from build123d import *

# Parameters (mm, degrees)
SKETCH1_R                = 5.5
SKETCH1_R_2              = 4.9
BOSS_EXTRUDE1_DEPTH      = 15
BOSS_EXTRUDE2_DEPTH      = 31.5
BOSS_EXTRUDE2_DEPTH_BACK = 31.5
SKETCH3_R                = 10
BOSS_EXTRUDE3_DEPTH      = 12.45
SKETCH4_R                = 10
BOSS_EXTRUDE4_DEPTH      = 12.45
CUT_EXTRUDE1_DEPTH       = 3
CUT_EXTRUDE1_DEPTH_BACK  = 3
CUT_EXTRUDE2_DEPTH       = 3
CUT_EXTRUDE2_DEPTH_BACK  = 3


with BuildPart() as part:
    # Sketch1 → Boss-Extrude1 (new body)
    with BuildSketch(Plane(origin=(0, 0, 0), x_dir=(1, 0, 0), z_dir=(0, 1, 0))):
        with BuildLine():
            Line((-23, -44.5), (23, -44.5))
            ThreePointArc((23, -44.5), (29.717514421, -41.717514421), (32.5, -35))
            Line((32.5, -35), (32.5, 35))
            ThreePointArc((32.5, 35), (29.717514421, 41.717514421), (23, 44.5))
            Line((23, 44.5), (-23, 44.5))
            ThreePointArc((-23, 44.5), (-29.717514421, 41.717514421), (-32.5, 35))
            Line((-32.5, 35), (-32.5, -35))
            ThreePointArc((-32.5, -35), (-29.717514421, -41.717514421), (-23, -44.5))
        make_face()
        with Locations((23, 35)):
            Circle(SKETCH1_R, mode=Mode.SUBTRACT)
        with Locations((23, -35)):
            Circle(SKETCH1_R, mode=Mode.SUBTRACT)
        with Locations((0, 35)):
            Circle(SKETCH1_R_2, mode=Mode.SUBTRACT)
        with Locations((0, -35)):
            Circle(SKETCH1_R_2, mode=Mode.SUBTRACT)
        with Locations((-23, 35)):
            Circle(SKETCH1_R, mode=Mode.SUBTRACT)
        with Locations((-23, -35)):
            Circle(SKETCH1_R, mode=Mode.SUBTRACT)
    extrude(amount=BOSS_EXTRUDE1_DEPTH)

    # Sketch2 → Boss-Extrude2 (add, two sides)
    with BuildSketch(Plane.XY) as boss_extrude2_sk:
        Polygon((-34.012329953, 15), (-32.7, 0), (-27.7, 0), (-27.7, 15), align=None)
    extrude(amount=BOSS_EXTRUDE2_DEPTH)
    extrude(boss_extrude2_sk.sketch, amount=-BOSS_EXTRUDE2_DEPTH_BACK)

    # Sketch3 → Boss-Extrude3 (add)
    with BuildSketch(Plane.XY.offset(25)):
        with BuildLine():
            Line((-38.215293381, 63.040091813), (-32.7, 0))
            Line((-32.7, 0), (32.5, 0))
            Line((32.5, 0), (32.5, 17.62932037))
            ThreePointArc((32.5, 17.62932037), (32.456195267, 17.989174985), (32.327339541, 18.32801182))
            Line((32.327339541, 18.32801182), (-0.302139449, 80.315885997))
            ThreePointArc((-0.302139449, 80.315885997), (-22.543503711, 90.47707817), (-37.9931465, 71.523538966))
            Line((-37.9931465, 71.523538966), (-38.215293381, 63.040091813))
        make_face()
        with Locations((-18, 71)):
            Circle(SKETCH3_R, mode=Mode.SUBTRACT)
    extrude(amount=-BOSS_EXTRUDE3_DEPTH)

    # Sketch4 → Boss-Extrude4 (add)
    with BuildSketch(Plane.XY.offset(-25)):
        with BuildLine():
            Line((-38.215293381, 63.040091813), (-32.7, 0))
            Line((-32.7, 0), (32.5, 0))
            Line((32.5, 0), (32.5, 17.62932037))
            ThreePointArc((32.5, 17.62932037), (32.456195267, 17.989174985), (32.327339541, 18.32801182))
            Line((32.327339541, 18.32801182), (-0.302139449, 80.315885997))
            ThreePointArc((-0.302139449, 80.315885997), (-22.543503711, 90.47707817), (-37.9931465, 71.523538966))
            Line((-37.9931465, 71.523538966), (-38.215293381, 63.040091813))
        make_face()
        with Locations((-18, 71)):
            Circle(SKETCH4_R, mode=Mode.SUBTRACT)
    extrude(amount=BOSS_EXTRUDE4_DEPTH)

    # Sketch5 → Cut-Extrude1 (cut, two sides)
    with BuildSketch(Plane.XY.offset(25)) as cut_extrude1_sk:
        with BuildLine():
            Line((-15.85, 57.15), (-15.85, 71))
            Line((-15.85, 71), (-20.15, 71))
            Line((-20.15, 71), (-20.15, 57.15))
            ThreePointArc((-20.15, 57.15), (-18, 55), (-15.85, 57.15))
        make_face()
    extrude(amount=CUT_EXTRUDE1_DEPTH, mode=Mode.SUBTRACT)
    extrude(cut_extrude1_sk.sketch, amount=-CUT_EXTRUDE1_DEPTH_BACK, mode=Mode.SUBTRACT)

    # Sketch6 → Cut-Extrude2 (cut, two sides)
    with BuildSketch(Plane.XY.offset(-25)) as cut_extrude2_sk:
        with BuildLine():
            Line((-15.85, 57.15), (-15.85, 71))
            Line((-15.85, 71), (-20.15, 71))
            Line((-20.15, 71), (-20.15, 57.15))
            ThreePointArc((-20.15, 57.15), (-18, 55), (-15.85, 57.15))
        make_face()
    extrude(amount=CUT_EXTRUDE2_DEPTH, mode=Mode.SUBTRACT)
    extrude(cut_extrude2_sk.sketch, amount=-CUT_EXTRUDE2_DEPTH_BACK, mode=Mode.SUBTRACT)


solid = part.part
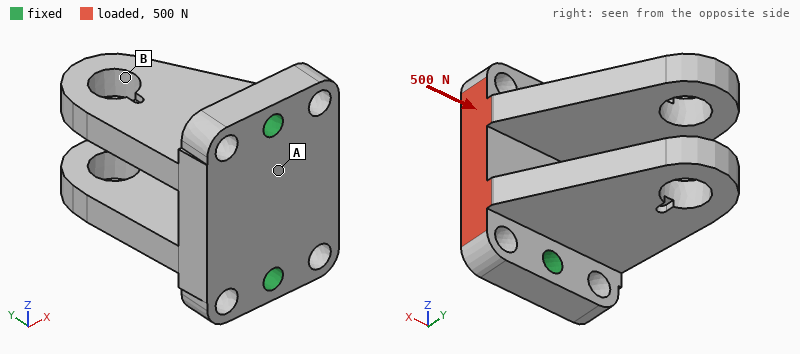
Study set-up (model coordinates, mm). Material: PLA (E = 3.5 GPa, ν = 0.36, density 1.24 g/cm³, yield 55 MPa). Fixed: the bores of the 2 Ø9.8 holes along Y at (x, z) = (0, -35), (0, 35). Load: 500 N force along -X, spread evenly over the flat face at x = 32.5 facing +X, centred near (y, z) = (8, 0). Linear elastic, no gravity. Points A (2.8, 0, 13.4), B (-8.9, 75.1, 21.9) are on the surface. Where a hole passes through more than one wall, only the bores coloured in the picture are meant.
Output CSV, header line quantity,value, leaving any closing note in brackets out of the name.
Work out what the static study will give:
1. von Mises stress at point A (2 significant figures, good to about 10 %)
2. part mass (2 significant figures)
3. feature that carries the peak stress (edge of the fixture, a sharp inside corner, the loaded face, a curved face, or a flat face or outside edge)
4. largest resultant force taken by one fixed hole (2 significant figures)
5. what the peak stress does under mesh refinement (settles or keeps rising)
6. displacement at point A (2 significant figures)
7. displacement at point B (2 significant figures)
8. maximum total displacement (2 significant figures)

quantity,value
von Mises stress at point A,0.29 MPa
part mass,200 g
feature that carries the peak stress,edge of the fixture
largest resultant force taken by one fixed hole,250 N
what the peak stress does under mesh refinement,keeps rising
displacement at point A,4.7 µm
displacement at point B,6.9 µm
maximum total displacement,8.4 µm
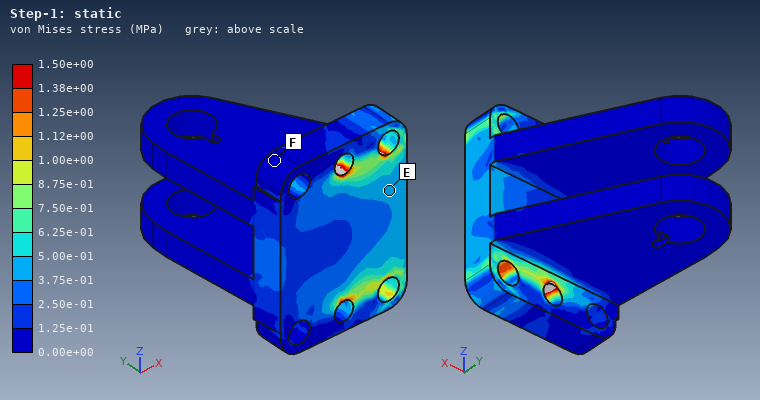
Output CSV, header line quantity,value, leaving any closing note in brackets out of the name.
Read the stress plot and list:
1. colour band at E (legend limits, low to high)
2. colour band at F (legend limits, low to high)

quantity,value
colour band at E,3.75e-01 to 5.00e-01 MPa
colour band at F,0.00e+00 to 1.25e-01 MPa
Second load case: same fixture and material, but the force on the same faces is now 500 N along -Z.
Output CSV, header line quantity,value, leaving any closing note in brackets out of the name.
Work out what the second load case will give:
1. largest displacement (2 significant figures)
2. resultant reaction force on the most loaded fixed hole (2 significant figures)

quantity,value
largest displacement,16 µm
resultant reaction force on the most loaded fixed hole,330 N
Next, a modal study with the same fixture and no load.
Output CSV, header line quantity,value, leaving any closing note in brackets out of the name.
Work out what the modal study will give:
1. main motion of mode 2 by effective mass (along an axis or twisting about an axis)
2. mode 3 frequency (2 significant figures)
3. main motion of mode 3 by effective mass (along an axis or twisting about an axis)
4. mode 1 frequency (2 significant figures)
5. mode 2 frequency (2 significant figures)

quantity,value
main motion of mode 2 by effective mass,along Z
mode 3 frequency,830 Hz
main motion of mode 3 by effective mass,along X
mode 1 frequency,650 Hz
mode 2 frequency,720 Hz
